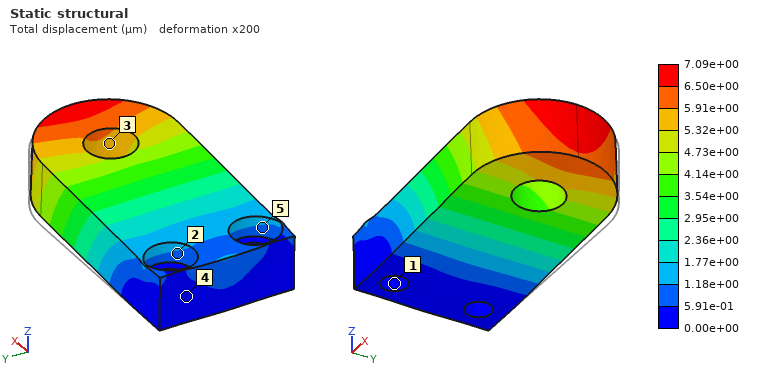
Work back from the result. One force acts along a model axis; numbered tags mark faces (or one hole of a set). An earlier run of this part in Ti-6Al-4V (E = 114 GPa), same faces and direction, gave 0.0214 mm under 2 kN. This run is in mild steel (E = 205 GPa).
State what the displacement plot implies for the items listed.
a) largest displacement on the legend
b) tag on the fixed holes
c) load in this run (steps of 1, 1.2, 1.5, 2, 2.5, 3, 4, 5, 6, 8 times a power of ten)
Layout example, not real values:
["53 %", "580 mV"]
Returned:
["7.09e+00 µm", "1", "1.2 kN"]
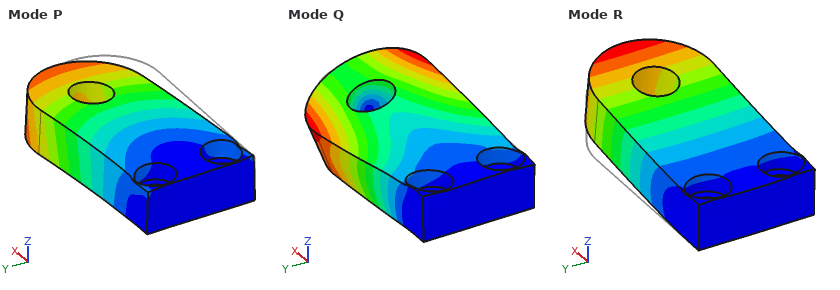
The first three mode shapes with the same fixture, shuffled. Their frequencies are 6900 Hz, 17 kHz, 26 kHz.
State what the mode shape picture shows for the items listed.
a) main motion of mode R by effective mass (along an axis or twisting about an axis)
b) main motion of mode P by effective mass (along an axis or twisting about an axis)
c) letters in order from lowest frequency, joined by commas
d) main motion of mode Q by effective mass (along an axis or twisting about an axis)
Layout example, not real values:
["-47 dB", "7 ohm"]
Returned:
["along Z", "along Y", "R, P, Q", "twisting about X"]
